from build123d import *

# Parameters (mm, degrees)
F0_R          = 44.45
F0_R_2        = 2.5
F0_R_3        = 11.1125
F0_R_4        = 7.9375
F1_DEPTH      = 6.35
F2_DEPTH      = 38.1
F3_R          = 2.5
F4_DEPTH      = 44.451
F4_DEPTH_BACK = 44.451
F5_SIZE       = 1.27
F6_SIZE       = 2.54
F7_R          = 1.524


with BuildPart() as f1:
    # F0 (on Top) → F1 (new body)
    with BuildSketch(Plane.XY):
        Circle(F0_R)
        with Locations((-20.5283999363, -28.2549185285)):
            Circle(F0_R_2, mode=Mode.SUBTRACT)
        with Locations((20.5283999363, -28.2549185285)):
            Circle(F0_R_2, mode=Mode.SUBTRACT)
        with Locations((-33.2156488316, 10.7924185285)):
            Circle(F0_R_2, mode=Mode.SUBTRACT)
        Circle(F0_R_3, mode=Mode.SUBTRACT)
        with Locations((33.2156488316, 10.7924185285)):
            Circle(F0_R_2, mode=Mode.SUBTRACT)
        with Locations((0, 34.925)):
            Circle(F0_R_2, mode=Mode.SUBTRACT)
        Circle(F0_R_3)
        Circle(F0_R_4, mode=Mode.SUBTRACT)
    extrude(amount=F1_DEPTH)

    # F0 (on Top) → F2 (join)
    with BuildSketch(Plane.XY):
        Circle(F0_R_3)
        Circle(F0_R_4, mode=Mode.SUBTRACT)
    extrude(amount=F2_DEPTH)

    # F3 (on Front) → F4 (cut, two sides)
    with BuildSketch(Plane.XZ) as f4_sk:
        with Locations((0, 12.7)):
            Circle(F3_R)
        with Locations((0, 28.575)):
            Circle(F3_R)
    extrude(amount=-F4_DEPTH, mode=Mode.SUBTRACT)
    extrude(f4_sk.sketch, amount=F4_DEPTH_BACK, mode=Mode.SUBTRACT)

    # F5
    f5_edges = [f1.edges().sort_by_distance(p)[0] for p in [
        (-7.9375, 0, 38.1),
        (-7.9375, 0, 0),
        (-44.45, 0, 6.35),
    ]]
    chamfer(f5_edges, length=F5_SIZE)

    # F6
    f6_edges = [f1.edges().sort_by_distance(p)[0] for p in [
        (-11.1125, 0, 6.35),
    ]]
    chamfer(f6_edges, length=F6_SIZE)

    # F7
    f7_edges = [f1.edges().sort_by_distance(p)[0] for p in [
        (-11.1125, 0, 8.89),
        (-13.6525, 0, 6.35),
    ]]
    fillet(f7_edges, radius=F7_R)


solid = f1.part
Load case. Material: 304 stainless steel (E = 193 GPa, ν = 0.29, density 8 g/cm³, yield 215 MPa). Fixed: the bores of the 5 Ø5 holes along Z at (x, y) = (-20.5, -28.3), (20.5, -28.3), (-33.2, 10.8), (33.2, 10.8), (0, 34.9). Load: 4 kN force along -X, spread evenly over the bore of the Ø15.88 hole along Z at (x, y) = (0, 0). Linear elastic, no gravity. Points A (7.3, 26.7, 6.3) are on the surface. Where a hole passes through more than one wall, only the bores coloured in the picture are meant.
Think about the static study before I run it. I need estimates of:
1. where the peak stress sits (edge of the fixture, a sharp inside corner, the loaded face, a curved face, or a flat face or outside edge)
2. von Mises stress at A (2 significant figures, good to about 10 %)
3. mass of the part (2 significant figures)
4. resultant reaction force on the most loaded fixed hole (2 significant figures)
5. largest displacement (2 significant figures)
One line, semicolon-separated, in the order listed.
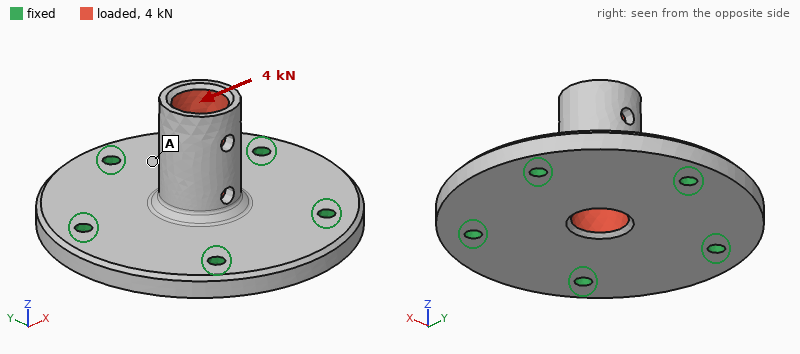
a curved face; 13 MPa; 350 g; 1.4 kN; 42 µm
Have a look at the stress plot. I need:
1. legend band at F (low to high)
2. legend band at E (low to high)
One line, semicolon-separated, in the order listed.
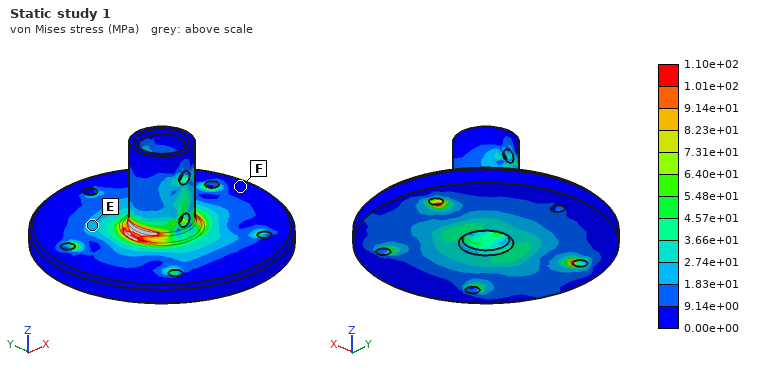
0.00e+00 to 9.14e+00 MPa; 1.83e+01 to 2.74e+01 MPa
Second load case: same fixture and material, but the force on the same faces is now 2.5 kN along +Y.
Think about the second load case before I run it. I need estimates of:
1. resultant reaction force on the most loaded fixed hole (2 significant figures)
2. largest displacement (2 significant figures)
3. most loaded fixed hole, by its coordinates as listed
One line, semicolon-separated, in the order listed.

920 N; 27 µm; (0, 34.9)
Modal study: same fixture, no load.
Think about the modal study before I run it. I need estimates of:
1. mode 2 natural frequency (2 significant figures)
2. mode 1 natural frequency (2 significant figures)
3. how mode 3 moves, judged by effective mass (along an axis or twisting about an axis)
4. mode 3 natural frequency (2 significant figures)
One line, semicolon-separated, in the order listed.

7400 Hz; 7400 Hz; along Z; 8100 Hz
